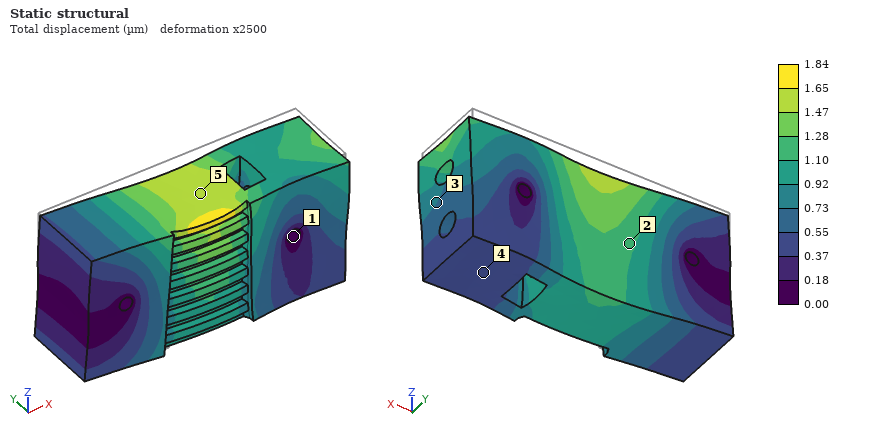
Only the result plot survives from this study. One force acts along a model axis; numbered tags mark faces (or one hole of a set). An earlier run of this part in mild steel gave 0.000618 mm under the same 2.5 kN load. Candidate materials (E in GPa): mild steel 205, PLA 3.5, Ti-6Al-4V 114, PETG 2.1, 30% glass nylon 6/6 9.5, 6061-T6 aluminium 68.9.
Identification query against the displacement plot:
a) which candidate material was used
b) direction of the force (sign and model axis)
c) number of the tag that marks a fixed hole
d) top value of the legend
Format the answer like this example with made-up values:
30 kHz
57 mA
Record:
6061-T6 aluminium
-Z
1
1.84 µm
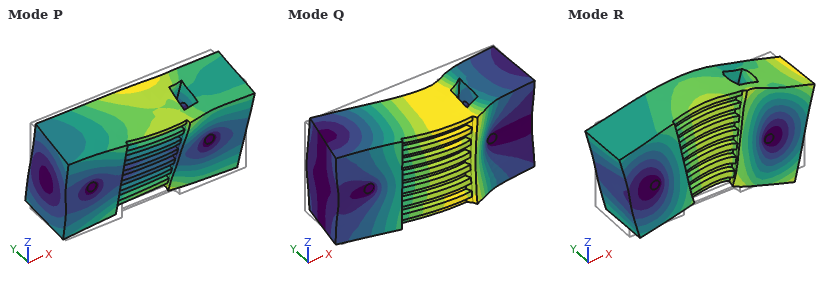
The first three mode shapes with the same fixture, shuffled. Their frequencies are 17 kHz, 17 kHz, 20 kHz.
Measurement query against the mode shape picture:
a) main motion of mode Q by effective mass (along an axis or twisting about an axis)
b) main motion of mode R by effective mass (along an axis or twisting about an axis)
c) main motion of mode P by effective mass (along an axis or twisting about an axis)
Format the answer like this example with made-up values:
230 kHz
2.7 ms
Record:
along Y
along Z
twisting about X
